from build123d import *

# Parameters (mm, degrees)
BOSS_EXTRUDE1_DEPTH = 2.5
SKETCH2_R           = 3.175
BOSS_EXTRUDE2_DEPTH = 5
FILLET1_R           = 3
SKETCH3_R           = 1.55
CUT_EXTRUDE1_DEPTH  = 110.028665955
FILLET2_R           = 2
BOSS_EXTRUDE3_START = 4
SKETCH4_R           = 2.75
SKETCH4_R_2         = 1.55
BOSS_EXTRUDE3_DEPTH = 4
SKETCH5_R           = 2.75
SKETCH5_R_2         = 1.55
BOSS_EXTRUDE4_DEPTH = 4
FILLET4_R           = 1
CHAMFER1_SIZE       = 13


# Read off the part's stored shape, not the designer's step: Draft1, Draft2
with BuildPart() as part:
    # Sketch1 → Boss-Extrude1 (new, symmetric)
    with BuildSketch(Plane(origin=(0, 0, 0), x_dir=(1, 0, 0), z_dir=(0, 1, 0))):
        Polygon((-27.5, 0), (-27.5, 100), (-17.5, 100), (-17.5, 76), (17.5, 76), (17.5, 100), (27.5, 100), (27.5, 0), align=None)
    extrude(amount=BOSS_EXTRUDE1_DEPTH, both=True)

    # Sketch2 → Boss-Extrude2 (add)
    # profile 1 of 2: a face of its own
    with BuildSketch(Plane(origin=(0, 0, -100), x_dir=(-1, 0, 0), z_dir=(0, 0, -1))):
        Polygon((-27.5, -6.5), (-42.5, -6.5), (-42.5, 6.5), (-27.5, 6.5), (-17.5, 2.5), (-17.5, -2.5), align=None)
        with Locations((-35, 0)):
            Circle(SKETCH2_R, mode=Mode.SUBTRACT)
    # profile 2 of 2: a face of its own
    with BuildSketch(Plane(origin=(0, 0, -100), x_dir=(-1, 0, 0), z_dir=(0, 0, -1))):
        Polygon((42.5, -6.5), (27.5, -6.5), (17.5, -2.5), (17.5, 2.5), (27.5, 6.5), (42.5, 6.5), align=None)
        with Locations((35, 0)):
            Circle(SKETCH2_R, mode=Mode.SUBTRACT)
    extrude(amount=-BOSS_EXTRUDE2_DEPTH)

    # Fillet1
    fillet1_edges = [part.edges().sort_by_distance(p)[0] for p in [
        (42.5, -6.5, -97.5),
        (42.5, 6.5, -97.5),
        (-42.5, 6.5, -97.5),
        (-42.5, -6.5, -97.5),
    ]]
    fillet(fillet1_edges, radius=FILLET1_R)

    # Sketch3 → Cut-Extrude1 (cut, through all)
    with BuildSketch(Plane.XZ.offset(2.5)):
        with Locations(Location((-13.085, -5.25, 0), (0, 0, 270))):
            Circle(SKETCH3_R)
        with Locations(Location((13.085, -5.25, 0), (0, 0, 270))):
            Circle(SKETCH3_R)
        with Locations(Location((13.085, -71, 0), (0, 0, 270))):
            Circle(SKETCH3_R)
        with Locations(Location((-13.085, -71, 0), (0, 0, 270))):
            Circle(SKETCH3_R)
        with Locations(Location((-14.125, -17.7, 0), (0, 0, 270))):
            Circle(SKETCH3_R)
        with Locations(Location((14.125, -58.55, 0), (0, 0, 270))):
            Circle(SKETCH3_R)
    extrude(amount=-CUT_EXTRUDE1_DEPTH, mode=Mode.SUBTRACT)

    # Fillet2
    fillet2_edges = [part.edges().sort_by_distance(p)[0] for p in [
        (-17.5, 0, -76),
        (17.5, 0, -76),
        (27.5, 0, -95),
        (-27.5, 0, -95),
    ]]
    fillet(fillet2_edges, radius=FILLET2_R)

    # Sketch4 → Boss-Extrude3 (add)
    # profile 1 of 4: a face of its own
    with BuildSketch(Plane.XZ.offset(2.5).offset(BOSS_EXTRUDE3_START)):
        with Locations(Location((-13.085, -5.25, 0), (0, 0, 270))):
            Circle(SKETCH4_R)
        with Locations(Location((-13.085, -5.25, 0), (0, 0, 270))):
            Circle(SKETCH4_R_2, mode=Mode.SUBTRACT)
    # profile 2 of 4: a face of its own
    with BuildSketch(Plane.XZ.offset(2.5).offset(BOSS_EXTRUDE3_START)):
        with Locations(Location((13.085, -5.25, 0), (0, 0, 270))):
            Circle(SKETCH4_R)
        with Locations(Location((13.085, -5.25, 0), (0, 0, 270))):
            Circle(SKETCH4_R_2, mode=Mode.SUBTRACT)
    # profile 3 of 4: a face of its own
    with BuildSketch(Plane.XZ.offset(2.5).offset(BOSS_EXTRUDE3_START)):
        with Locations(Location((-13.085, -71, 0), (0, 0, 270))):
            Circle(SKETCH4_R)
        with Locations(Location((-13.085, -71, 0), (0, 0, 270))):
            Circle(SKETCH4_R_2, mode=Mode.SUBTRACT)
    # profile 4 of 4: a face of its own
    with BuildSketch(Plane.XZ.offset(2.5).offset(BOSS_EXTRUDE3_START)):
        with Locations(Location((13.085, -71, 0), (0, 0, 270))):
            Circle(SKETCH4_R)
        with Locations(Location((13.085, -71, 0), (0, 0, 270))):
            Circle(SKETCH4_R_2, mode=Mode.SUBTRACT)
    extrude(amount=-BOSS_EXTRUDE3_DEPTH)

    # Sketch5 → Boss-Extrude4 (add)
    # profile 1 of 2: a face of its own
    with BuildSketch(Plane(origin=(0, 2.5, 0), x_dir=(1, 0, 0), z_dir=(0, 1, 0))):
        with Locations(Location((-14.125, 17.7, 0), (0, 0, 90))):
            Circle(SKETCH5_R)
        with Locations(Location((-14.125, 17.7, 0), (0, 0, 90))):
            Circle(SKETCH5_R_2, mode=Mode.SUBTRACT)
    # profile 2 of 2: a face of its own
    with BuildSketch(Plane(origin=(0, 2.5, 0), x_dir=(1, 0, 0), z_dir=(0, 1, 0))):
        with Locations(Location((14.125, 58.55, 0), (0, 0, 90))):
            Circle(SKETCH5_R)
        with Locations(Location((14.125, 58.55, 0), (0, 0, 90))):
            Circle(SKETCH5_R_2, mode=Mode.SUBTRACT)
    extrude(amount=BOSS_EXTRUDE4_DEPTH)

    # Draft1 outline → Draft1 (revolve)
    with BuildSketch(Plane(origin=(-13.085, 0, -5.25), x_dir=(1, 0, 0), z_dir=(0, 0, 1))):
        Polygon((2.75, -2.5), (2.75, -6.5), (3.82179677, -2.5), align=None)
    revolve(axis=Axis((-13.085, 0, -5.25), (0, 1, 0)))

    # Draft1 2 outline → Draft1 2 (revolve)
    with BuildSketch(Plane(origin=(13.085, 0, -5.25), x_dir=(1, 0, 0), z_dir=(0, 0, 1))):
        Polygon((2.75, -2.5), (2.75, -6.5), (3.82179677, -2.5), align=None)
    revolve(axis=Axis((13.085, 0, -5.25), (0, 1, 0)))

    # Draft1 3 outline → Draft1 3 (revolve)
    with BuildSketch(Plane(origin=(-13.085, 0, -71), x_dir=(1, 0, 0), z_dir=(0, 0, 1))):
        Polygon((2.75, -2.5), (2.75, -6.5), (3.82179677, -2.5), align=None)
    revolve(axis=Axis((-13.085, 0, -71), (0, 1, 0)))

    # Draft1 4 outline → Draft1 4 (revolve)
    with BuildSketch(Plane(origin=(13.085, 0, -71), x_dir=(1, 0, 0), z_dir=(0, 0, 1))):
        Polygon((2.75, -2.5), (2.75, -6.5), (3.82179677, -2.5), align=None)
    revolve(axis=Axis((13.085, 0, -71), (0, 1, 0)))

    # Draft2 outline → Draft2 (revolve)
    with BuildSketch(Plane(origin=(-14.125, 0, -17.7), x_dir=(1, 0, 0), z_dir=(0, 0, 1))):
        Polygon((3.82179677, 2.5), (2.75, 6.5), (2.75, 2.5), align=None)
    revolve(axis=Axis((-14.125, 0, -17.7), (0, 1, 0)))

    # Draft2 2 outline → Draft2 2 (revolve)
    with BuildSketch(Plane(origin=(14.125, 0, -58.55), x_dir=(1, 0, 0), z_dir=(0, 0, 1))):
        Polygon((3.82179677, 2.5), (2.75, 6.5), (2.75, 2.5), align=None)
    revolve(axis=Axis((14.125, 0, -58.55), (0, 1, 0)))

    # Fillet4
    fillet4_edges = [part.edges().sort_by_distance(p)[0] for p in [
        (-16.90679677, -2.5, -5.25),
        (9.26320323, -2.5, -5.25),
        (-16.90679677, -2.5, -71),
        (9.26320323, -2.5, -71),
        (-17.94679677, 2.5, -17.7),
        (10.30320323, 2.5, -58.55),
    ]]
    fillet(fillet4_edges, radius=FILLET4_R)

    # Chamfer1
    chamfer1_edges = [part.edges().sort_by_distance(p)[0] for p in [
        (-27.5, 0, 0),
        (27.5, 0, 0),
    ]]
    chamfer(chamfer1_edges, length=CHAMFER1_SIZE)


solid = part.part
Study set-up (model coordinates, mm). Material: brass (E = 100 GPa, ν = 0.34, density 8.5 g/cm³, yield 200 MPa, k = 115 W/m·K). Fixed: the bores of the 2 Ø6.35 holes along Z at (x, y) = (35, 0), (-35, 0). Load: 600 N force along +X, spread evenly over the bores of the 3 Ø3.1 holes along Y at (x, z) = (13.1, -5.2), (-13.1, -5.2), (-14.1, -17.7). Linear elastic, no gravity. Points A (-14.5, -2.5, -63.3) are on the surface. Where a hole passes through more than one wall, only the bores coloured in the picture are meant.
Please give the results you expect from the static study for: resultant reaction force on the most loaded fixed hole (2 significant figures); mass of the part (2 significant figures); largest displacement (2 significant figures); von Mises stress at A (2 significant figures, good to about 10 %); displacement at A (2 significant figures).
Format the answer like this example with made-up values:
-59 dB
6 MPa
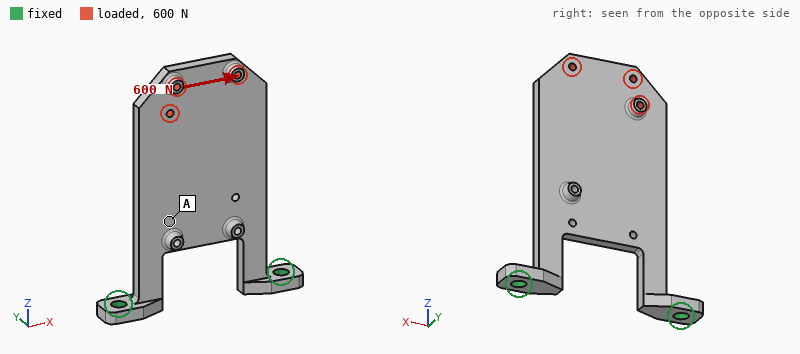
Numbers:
970 N
210 g
64 µm
10 MPa
19 µm
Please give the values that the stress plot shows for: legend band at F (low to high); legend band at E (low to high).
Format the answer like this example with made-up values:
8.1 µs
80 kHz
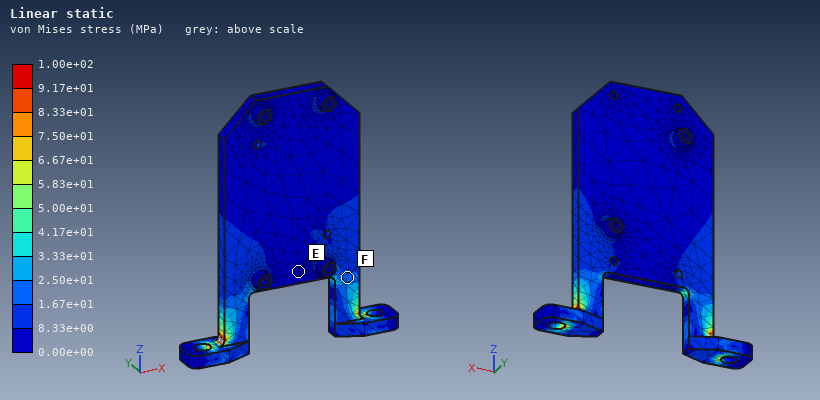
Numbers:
1.67e+01 to 2.50e+01 MPa
0.00e+00 to 8.33e+00 MPa
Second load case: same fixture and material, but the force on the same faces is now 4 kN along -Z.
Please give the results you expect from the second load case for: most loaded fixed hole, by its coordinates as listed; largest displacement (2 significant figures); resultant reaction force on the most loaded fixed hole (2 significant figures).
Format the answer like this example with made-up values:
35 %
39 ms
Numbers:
(-35, 0)
0.46 mm
2.4 kN
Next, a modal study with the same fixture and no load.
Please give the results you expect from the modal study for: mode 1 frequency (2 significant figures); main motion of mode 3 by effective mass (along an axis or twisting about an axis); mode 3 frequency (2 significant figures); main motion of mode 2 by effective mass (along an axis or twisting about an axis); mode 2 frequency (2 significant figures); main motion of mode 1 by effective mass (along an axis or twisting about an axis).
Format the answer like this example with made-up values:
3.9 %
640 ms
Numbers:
190 Hz
along Y
1500 Hz
twisting about Z
1000 Hz
along Y
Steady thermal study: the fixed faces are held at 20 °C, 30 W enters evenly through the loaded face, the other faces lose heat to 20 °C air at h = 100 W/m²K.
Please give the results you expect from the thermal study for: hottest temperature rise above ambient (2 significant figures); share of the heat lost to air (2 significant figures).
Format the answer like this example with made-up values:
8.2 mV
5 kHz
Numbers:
50 K
85 %
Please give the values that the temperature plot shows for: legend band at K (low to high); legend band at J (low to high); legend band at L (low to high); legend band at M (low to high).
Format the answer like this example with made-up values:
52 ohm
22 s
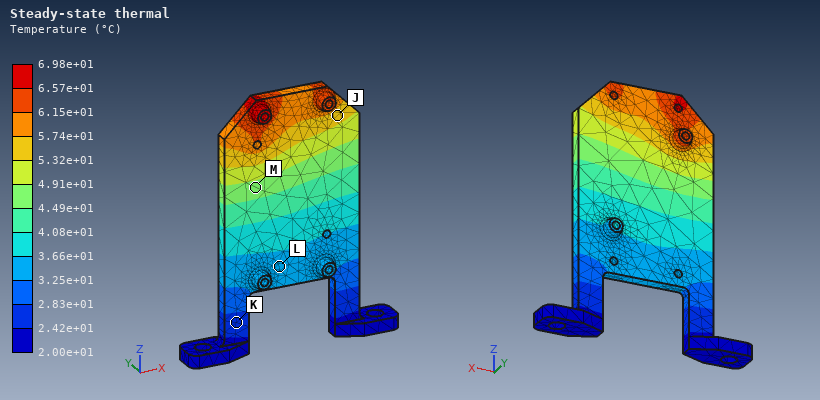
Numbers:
2.42e+01 to 2.83e+01 °C
5.32e+01 to 5.74e+01 °C
3.25e+01 to 3.66e+01 °C
4.49e+01 to 4.91e+01 °C
